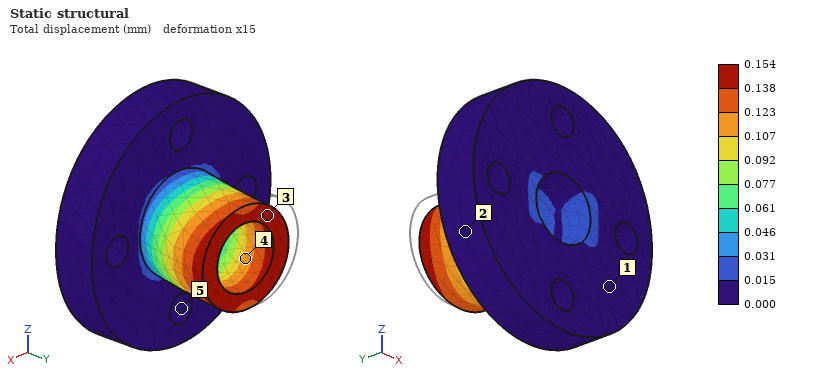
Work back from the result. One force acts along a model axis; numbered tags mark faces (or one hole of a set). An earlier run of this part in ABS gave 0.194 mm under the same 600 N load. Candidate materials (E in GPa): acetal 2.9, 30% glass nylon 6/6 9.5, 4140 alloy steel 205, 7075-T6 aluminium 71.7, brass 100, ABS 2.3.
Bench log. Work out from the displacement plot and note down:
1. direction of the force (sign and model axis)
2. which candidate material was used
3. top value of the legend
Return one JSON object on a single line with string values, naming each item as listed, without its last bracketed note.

{"direction of the force": "+X", "which candidate material was used": "acetal", "top value of the legend": "0.154 mm"}
